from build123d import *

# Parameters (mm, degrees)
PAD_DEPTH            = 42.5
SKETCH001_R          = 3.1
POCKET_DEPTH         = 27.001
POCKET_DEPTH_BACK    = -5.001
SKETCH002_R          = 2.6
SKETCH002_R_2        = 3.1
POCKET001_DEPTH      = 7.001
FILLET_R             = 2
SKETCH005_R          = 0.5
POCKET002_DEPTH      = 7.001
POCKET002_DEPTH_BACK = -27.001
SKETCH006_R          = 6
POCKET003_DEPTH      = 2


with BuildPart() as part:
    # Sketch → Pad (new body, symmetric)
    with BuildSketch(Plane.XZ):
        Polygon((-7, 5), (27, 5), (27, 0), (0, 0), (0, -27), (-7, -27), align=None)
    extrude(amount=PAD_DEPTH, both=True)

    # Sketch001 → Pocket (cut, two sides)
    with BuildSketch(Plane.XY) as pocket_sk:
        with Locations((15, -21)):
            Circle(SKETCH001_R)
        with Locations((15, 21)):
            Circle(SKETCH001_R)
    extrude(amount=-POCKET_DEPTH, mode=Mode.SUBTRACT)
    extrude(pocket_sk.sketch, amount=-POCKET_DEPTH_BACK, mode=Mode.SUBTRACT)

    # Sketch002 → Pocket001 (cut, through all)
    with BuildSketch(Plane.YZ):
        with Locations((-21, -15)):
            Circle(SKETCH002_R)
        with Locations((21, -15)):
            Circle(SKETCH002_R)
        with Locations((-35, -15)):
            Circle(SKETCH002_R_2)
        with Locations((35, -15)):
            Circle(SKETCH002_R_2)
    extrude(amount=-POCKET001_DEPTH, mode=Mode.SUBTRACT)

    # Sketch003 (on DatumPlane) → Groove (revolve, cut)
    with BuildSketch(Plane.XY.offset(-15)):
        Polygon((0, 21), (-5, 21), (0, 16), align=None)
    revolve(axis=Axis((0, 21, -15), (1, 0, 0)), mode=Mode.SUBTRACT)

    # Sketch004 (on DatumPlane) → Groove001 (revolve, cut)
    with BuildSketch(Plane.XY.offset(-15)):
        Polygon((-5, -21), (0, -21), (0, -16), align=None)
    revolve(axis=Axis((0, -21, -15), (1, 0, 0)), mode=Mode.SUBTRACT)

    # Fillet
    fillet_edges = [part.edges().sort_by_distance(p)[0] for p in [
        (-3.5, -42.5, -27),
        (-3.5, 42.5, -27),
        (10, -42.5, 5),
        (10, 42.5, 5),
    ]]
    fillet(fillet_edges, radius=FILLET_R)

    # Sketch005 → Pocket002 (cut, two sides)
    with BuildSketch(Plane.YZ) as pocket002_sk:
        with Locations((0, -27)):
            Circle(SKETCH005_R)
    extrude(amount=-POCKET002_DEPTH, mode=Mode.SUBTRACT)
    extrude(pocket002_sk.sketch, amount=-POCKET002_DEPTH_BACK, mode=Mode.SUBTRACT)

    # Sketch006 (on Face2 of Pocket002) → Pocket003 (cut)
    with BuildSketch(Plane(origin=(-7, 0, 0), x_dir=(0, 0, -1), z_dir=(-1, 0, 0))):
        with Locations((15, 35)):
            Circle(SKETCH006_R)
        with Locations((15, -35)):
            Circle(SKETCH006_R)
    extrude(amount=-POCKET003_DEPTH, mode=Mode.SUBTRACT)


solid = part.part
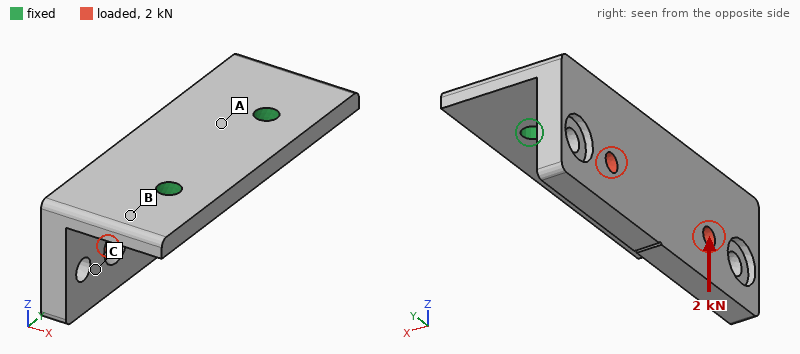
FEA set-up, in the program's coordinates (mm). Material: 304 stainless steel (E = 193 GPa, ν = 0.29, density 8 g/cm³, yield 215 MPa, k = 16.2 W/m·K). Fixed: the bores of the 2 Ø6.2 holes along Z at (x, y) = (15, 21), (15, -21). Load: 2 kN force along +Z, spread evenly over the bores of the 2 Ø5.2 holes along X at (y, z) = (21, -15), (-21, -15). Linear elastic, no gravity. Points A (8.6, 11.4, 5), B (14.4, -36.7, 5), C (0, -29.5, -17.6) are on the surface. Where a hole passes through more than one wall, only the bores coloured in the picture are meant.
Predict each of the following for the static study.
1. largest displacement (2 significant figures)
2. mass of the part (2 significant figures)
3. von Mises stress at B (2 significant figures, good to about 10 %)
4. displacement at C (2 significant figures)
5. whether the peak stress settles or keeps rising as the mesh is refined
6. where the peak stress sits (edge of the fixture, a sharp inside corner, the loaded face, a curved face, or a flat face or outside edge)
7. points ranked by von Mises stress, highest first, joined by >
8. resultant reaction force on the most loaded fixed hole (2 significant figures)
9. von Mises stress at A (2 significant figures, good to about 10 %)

87 µm
230 g
39 MPa
57 µm
keeps rising
edge of the fixture
A > B > C
1.0 kN
63 MPa
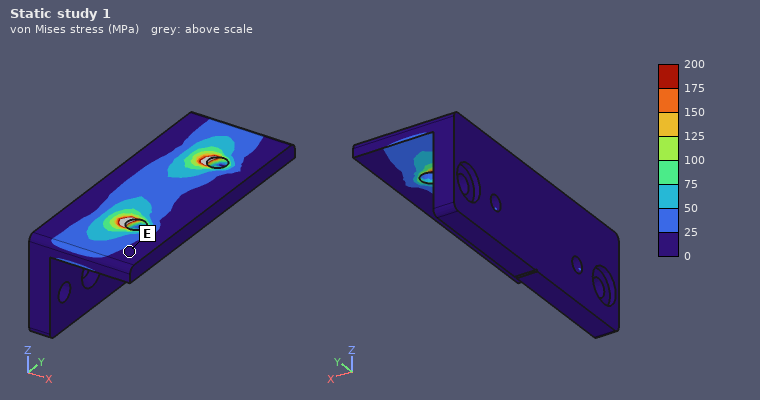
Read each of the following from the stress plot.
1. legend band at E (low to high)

0 to 25 MPa
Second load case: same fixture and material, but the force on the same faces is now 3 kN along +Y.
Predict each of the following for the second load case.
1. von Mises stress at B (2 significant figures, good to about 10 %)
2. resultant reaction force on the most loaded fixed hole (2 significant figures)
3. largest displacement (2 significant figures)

27 MPa
2.2 kN
41 µm
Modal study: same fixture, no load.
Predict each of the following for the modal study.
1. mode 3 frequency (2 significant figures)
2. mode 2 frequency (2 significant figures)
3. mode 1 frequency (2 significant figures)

6100 Hz
3400 Hz
2000 Hz
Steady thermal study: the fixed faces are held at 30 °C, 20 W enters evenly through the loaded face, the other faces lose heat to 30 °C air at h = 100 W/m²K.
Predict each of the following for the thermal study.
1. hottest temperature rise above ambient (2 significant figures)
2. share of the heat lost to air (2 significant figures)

52 K
84 %
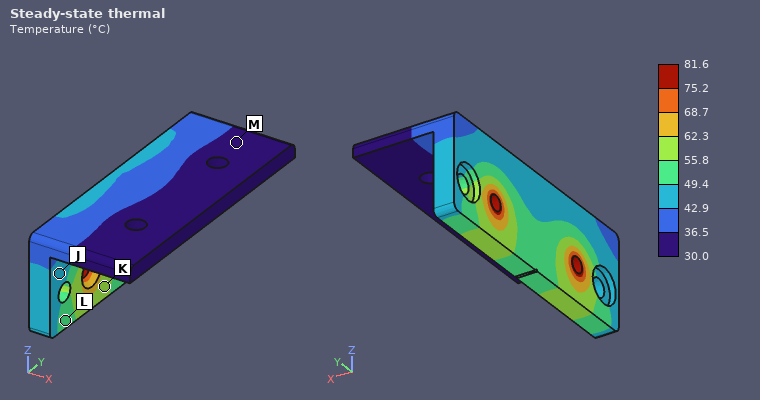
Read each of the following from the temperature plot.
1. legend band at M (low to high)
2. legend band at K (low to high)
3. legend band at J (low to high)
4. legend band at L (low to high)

30.0 to 36.5 °C
55.8 to 62.3 °C
42.9 to 49.4 °C
49.4 to 55.8 °C
